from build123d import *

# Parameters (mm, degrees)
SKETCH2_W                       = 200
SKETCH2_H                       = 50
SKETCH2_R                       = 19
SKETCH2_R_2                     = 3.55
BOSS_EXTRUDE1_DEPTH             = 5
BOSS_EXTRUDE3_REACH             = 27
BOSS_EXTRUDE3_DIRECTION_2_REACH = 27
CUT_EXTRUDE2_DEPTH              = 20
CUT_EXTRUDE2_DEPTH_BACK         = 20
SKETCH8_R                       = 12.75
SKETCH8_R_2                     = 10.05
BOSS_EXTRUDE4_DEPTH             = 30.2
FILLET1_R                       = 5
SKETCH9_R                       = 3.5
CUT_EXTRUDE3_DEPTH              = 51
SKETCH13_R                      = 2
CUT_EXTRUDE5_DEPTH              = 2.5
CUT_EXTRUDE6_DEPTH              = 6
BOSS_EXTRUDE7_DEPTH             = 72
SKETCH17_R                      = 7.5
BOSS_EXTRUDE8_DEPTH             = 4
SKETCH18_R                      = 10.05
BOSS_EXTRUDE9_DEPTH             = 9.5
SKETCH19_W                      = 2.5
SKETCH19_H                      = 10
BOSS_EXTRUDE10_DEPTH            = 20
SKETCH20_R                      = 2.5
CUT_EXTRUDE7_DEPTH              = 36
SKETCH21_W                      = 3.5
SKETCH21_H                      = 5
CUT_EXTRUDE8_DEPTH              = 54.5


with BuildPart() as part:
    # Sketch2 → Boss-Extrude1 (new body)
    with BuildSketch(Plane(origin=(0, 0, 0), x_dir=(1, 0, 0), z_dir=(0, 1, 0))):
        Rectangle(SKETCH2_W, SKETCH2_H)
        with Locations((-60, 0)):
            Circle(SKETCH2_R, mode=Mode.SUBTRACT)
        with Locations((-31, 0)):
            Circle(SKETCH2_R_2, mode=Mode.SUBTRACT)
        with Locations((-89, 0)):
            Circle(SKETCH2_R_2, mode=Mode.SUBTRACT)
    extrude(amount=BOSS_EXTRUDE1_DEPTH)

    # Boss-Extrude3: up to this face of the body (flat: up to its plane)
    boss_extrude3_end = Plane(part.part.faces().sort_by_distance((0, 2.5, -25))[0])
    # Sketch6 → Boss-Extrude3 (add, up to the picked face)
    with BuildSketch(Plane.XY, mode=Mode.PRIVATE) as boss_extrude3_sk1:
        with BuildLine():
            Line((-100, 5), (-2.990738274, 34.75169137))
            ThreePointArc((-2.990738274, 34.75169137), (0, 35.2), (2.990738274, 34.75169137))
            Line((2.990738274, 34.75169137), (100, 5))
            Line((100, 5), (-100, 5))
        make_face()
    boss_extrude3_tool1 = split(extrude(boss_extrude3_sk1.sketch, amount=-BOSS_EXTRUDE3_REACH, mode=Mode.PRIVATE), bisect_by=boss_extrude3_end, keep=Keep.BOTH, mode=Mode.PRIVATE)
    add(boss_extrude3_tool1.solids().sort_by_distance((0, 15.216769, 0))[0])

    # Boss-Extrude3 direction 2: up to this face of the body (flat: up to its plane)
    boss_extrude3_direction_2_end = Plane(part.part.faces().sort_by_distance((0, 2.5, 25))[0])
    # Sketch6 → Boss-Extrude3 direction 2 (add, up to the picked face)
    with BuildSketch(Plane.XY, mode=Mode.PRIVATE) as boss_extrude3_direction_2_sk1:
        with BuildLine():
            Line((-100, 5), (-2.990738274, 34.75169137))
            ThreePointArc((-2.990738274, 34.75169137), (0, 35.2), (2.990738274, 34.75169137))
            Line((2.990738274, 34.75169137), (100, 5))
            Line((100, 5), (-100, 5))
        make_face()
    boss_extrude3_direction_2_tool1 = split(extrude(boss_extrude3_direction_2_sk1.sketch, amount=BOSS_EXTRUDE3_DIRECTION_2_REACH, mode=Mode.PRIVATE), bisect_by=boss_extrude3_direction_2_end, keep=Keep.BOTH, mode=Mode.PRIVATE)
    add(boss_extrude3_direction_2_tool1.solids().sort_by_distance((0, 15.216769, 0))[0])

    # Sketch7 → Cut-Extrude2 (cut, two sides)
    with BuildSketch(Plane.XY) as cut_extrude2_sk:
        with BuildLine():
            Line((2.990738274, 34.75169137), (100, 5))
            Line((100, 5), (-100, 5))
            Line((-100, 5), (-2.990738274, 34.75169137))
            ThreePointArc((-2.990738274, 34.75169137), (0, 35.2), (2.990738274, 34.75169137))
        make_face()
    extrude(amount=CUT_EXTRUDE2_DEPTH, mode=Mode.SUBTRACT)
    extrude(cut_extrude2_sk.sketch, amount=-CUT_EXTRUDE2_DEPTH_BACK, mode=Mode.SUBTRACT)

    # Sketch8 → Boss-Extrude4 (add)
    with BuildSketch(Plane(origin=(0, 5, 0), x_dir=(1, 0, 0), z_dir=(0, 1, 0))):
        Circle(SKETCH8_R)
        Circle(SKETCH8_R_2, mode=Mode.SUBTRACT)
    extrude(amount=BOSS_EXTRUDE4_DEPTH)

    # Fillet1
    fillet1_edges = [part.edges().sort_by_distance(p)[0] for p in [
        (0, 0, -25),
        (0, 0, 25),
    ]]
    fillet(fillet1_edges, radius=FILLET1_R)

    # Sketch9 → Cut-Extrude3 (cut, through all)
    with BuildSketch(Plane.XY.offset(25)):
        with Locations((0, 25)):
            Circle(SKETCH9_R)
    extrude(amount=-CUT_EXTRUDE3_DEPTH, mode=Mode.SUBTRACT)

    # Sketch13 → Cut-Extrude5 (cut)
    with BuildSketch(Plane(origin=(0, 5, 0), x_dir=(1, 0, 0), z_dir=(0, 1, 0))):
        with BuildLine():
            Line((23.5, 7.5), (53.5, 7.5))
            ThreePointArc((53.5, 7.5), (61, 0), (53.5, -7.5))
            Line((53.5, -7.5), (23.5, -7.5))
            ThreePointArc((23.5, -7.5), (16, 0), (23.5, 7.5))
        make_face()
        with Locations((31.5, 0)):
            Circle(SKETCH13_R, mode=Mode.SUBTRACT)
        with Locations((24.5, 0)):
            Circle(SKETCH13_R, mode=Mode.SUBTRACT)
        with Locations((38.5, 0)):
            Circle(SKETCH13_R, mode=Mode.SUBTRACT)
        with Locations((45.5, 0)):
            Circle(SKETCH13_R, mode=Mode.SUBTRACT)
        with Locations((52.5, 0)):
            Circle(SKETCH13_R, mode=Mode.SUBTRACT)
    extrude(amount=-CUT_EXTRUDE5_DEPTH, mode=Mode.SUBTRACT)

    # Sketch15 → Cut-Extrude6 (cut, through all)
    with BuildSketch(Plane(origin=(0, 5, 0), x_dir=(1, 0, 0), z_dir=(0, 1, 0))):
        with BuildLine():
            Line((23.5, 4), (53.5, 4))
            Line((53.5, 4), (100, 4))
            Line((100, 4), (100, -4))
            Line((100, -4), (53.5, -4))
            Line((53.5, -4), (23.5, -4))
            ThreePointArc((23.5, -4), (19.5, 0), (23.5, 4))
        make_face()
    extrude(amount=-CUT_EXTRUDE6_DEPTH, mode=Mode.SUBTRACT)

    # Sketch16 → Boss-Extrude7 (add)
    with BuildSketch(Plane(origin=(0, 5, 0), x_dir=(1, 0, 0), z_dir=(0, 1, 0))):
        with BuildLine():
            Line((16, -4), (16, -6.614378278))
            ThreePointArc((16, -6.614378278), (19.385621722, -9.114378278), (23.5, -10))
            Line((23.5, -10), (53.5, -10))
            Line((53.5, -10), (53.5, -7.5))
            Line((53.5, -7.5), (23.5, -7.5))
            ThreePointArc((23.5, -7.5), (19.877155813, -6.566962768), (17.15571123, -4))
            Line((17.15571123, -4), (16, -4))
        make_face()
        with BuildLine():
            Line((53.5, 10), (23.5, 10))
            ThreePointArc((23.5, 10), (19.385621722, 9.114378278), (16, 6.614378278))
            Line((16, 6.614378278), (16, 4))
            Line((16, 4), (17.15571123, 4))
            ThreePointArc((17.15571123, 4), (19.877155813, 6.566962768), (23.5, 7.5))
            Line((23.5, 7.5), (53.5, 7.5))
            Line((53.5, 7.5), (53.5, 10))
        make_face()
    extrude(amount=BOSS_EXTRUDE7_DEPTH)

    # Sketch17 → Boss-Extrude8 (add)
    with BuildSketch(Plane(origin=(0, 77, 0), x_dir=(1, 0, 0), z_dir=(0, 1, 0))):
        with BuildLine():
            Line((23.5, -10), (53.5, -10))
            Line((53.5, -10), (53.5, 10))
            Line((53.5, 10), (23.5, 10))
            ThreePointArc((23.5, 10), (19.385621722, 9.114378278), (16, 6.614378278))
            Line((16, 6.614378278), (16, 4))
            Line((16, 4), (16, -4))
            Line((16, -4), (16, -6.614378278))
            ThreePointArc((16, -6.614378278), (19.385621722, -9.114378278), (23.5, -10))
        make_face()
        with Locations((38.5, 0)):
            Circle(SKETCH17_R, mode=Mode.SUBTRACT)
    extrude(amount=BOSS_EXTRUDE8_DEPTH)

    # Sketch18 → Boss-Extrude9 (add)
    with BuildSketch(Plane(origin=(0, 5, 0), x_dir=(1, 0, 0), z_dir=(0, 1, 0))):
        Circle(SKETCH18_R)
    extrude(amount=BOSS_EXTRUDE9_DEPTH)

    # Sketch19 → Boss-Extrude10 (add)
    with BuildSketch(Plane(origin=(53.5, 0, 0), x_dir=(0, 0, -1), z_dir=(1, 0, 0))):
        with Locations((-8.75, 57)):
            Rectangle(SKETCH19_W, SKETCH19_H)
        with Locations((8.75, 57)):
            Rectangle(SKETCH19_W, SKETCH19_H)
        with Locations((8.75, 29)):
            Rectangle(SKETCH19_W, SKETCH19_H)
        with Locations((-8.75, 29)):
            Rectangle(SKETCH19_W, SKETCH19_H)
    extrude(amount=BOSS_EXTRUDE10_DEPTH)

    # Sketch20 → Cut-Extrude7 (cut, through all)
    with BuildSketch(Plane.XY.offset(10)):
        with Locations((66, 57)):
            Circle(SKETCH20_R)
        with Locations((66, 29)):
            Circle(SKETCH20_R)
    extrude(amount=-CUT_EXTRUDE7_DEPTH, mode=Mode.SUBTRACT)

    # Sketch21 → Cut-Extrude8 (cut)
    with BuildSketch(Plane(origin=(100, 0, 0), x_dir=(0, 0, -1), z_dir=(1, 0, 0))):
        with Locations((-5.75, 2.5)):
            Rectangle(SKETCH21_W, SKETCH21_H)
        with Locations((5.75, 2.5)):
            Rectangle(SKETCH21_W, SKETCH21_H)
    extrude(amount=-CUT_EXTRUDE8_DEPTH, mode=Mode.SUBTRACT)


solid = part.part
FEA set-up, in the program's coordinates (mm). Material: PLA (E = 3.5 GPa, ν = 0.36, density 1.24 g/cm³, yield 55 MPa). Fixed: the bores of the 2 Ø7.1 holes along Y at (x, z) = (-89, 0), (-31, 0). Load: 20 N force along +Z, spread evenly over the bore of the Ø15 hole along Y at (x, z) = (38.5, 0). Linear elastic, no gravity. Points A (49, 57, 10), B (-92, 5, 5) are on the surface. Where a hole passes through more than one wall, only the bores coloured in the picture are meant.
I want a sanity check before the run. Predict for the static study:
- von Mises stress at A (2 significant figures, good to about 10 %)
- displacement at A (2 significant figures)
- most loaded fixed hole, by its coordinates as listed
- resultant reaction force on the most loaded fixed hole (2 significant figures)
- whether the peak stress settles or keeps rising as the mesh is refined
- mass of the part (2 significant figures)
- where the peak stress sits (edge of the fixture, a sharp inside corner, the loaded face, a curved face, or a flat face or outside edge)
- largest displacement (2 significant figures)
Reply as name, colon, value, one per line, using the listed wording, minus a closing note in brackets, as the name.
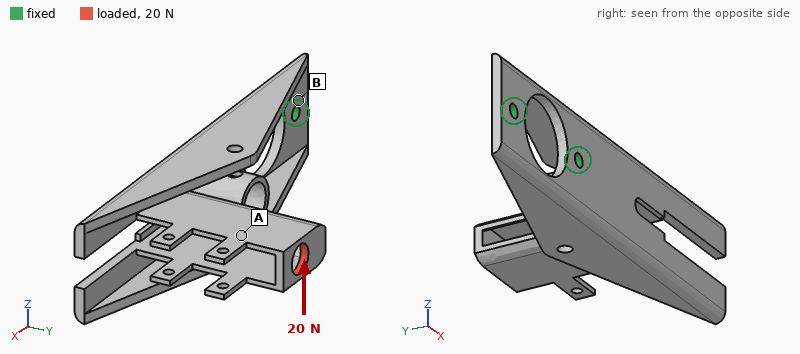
von Mises stress at A: 1.8 MPa
displacement at A: 1.9 mm
most loaded fixed hole, by its coordinates as listed: (-31, 0)
resultant reaction force on the most loaded fixed hole: 29 N
whether the peak stress settles or keeps rising as the mesh is refined: keeps rising
mass of the part: 120 g
where the peak stress sits: edge of the fixture
largest displacement: 2.6 mm
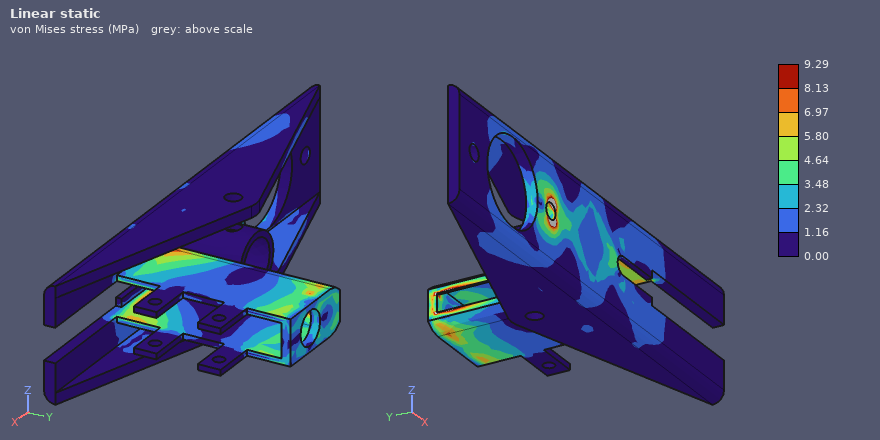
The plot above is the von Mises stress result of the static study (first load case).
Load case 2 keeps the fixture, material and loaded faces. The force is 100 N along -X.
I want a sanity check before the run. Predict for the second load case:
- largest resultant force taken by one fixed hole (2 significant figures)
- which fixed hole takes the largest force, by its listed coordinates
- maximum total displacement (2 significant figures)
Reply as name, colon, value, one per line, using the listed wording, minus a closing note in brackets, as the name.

largest resultant force taken by one fixed hole: 190 N
which fixed hole takes the largest force, by its listed coordinates: (-89, 0)
maximum total displacement: 2.3 mm
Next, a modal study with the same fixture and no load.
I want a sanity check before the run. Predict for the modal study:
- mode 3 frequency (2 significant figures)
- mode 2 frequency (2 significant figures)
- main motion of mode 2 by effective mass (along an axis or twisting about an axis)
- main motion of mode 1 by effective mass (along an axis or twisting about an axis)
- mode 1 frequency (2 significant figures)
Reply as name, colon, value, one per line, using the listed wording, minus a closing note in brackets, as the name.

mode 3 frequency: 330 Hz
mode 2 frequency: 210 Hz
main motion of mode 2 by effective mass: along Y
main motion of mode 1 by effective mass: along Z
mode 1 frequency: 140 Hz
